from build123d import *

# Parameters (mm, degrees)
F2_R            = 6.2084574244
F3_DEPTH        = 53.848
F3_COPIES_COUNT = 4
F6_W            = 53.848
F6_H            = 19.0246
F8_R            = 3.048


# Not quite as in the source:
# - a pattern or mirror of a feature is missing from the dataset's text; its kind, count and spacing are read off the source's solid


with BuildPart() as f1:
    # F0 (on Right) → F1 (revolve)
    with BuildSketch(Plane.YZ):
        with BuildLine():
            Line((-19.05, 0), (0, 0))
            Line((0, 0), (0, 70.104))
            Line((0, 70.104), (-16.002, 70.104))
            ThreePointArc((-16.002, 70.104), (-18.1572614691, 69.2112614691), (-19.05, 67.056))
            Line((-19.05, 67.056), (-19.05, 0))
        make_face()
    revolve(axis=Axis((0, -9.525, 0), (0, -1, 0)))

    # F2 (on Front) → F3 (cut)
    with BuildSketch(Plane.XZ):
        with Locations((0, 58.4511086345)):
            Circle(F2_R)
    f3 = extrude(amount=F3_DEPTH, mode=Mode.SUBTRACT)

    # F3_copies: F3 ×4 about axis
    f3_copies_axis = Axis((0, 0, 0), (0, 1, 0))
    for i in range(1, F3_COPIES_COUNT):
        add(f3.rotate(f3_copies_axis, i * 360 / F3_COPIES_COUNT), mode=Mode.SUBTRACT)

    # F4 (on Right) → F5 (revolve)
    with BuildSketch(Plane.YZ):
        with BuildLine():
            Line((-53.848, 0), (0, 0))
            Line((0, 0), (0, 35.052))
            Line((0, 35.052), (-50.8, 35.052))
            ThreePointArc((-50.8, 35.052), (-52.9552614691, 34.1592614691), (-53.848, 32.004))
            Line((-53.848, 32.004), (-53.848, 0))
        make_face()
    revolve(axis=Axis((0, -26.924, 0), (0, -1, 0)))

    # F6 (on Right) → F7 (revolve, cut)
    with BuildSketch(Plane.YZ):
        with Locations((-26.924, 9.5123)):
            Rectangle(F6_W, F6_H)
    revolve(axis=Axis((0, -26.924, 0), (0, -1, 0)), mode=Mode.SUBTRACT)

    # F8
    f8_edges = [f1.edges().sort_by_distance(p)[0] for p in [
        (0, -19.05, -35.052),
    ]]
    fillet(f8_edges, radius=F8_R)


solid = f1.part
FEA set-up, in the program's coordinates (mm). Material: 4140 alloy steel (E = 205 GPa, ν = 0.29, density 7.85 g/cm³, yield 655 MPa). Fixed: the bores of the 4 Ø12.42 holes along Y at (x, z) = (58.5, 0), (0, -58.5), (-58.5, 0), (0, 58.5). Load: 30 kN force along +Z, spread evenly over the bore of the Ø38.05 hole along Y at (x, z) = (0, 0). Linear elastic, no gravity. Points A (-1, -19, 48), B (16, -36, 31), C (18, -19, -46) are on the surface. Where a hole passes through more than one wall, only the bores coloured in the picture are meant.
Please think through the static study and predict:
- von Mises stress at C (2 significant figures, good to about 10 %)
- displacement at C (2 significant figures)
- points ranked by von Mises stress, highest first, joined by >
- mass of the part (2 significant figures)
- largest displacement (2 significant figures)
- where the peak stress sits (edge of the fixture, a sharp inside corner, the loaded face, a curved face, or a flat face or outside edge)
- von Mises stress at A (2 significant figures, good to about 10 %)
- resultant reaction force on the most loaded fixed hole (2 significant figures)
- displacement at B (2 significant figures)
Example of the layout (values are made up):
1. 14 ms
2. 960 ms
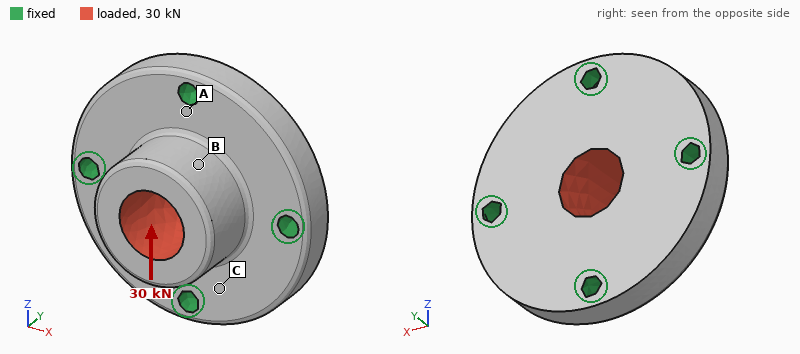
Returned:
1. 10 MPa
2. 1.8 µm
3. A > C > B
4. 2.8 kg
5. 9.6 µm
6. a curved face
7. 19 MPa
8. 11 kN
9. 6.7 µm
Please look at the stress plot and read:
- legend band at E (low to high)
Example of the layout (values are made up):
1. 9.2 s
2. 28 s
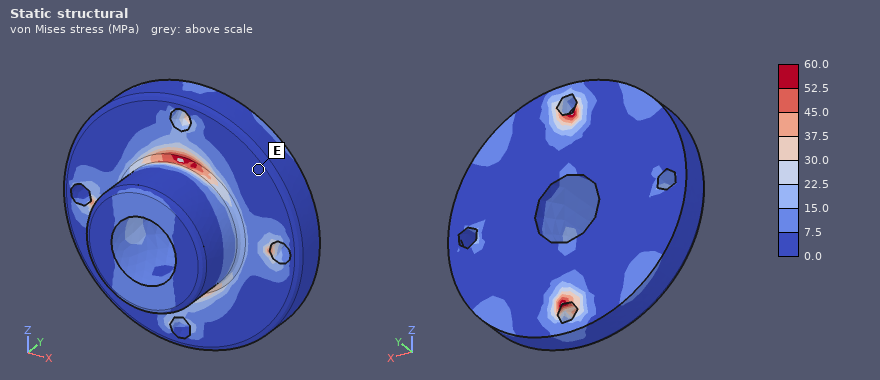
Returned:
1. 0.0 to 7.5 MPa
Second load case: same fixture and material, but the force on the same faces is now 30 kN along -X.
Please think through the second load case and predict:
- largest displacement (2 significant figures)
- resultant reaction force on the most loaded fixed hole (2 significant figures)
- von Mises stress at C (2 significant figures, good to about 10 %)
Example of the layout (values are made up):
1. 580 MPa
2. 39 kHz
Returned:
1. 9.6 µm
2. 11 kN
3. 6.9 MPa
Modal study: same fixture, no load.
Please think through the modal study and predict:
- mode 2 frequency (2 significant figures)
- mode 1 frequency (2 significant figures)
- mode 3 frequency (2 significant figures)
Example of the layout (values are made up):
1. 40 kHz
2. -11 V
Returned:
1. 8600 Hz
2. 8300 Hz
3. 8600 Hz
